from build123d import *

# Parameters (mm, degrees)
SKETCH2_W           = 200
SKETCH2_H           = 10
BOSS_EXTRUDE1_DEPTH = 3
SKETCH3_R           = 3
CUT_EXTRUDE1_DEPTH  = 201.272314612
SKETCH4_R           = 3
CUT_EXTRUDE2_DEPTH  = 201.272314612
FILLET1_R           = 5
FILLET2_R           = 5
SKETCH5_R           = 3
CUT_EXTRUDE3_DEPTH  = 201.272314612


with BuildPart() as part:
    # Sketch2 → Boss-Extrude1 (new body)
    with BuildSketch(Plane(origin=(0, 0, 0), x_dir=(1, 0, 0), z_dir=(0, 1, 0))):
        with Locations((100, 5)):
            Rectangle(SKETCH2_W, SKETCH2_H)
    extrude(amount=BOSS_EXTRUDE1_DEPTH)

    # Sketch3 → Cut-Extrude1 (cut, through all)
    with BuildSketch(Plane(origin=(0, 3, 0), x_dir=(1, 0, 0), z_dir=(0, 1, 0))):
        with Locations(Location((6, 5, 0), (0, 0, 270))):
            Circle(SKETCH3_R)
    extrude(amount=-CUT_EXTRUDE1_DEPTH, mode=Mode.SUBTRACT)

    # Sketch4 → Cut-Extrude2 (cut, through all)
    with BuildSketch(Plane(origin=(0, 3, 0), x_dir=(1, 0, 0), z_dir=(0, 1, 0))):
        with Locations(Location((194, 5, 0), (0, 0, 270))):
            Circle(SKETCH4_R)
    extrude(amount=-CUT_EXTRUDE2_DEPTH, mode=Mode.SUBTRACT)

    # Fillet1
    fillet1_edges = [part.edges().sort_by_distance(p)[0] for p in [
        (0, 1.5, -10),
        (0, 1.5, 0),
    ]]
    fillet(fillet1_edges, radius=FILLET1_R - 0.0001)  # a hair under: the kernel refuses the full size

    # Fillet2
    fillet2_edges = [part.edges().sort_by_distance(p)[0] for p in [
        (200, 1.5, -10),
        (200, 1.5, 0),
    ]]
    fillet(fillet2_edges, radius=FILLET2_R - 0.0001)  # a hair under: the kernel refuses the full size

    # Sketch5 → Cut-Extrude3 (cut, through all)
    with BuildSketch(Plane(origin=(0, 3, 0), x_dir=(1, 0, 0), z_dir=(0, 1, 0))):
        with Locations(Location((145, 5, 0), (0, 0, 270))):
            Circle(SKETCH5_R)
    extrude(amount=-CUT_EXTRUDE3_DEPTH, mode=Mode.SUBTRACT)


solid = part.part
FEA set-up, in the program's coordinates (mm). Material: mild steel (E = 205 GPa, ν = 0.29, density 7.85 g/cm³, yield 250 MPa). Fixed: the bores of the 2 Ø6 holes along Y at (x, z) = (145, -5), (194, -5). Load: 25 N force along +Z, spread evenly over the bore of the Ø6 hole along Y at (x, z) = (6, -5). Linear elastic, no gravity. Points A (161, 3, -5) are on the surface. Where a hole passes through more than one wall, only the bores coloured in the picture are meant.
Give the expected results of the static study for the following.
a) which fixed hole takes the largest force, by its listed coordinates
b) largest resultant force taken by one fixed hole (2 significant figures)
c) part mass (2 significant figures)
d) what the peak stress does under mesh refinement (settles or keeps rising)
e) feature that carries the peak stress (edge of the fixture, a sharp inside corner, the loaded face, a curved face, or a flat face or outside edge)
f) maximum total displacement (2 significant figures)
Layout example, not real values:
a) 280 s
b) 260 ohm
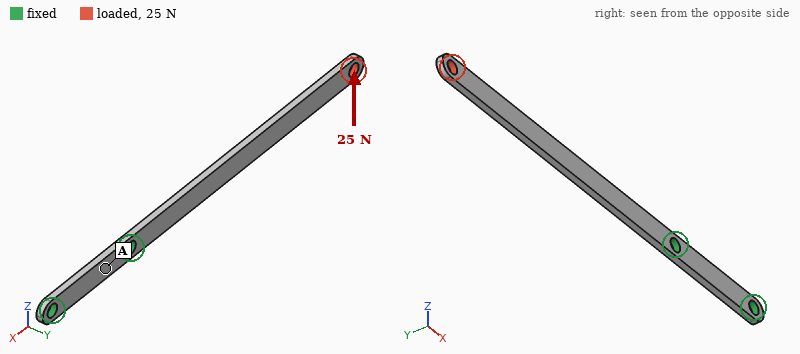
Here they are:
a) (145, -5)
b) 29 N
c) 45 g
d) keeps rising
e) edge of the fixture
f) 0.46 mm
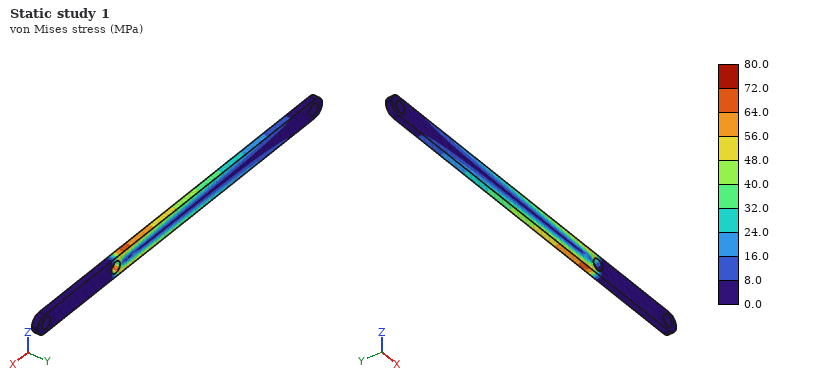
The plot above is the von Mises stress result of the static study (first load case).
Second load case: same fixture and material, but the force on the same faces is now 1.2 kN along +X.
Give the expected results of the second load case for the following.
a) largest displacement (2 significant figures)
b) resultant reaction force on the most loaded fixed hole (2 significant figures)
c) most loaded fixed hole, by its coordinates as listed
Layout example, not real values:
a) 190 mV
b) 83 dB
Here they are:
a) 30 µm
b) 1.2 kN
c) (145, -5)
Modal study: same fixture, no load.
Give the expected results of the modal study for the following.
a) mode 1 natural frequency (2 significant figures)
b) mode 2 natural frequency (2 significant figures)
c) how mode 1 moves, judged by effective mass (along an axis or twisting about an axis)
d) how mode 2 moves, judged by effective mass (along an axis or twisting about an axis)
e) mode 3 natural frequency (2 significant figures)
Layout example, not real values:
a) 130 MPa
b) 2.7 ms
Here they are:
a) 130 Hz
b) 410 Hz
c) along Y
d) along Z
e) 800 Hz
